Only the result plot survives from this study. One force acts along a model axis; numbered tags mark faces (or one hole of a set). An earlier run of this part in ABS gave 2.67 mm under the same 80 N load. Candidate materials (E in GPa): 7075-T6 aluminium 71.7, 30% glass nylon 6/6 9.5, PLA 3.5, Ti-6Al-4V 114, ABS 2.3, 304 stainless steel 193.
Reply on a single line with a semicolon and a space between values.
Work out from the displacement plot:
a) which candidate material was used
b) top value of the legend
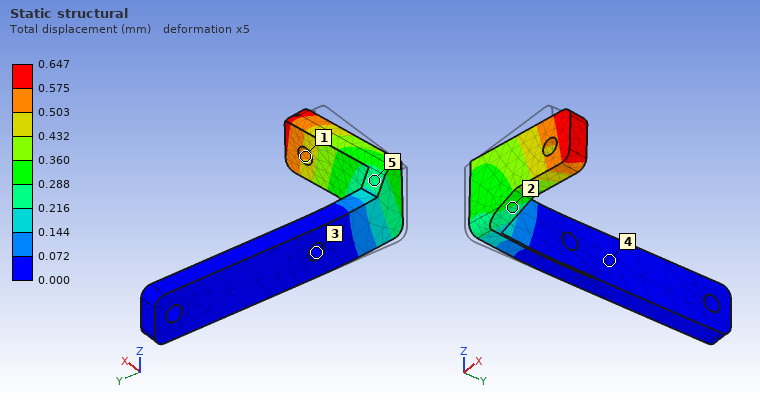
30% glass nylon 6/6; 0.647 mm
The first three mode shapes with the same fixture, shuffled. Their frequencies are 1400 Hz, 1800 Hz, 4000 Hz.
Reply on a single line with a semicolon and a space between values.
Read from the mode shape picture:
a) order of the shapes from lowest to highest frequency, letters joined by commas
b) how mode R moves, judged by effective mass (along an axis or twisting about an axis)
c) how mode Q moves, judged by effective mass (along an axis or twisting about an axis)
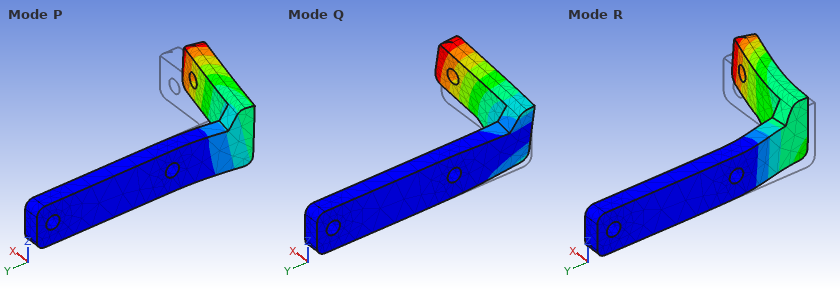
P, Q, R; along X; along Z
